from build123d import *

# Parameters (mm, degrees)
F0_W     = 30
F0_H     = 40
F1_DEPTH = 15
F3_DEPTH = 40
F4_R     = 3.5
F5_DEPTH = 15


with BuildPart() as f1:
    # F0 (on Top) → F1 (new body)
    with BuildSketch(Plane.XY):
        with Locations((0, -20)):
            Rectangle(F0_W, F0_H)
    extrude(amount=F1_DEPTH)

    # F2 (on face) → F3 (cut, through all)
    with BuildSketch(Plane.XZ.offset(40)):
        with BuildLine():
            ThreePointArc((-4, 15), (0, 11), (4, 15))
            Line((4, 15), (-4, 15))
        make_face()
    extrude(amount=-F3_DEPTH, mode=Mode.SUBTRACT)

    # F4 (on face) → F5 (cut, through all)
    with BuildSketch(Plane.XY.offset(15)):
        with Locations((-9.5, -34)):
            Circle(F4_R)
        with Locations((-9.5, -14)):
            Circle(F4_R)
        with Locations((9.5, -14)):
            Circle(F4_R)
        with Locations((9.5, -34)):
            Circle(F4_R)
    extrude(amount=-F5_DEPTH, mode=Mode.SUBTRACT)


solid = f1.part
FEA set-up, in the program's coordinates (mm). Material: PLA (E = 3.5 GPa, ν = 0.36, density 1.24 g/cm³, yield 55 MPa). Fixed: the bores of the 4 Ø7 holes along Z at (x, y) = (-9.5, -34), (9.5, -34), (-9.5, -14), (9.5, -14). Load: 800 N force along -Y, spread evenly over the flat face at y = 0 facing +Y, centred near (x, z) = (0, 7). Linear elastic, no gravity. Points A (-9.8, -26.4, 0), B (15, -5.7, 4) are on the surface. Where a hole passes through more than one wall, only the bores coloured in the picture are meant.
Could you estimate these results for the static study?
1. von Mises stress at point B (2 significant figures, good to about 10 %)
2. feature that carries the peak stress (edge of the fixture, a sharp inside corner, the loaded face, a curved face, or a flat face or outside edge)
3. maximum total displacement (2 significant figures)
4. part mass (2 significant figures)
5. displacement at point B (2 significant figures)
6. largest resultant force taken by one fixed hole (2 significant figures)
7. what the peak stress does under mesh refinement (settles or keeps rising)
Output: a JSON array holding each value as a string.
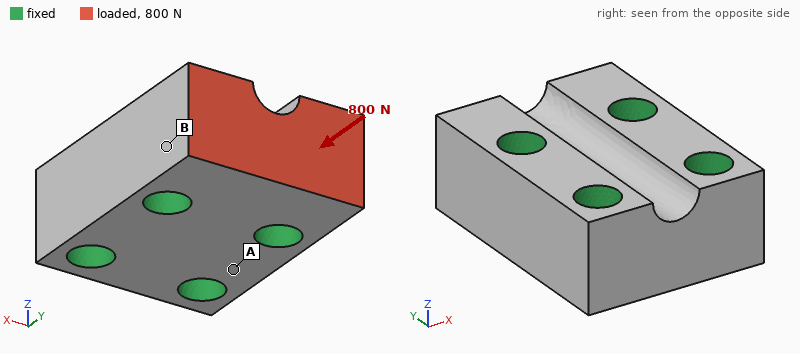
["1.6 MPa", "edge of the fixture", "7.6 µm", "18 g", "4.5 µm", "390 N", "keeps rising"]
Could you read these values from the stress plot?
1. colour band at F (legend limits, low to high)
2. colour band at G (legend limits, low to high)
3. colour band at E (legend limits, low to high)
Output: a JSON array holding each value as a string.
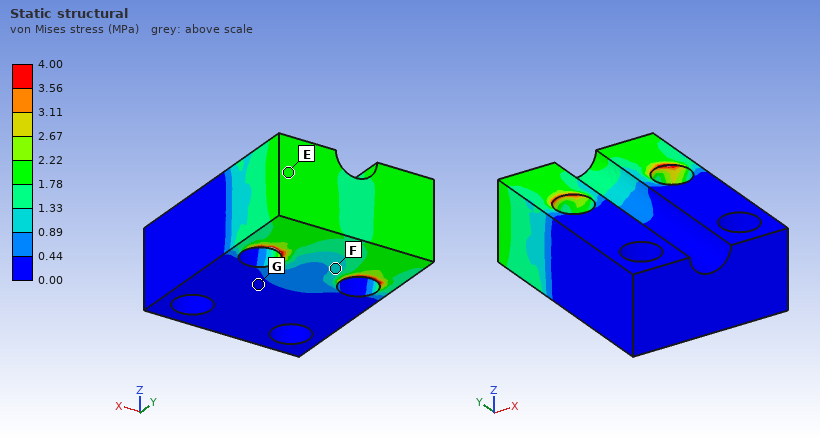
["0.89 to 1.33 MPa", "0.00 to 0.44 MPa", "1.78 to 2.22 MPa"]
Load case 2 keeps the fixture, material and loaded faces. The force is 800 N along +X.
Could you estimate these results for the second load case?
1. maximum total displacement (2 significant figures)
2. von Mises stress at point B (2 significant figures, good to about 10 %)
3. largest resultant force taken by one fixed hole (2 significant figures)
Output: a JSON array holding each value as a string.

["37 µm", "3.4 MPa", "550 N"]
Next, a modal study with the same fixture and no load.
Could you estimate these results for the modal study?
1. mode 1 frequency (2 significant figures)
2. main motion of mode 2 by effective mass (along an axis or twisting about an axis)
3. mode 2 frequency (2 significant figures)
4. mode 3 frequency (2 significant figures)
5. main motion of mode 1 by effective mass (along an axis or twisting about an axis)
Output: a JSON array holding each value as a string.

["16 kHz", "along X", "17 kHz", "19 kHz", "along Z"]
